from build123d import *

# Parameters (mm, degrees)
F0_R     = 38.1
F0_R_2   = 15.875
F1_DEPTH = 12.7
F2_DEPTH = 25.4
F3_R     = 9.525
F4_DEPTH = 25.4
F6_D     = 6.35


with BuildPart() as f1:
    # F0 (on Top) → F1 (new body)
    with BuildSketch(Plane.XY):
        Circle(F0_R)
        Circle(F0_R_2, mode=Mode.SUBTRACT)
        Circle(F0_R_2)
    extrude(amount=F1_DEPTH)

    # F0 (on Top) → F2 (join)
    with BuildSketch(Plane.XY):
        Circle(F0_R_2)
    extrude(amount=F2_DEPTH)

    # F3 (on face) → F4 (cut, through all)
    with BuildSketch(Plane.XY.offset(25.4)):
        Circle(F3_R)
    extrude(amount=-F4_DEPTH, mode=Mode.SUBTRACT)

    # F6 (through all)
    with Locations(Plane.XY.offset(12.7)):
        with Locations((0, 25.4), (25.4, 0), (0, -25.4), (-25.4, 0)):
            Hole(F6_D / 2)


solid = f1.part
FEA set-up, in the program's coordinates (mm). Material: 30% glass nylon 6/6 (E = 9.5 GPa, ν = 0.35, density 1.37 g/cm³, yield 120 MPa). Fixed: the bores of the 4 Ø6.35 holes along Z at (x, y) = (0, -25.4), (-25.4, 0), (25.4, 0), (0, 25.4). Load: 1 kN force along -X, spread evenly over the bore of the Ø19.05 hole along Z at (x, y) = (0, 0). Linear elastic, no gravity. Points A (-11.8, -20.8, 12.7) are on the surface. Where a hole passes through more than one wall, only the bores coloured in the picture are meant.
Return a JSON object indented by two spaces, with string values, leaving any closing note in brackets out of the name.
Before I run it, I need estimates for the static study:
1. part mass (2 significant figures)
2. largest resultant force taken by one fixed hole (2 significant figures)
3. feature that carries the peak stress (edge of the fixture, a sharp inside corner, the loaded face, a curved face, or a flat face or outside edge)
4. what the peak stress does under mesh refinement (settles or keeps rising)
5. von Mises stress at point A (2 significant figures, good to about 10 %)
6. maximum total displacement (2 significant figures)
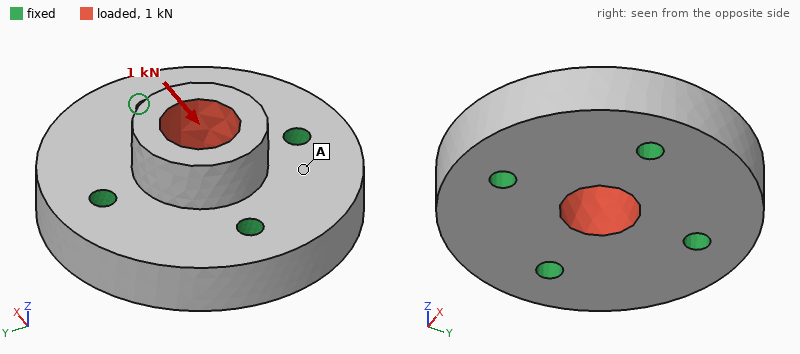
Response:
{
  "part mass": "81 g",
  "largest resultant force taken by one fixed hole": "340 N",
  "feature that carries the peak stress": "edge of the fixture",
  "what the peak stress does under mesh refinement": "keeps rising",
  "von Mises stress at point A": "0.44 MPa",
  "maximum total displacement": "8.9 µm"
}
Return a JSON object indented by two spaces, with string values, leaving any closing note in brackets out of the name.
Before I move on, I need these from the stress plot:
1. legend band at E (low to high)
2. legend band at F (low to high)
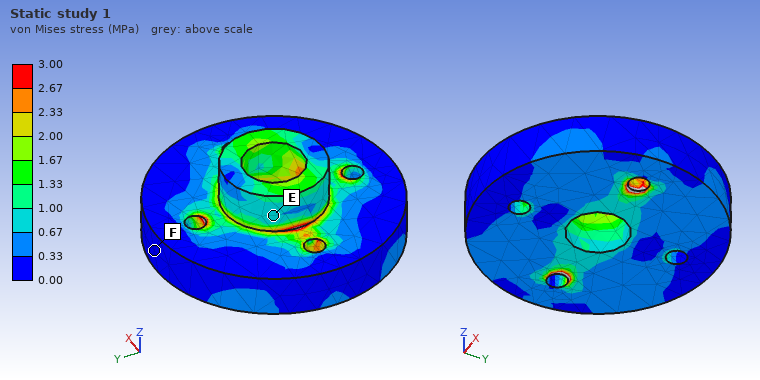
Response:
{
  "legend band at E": "0.67 to 1.00 MPa",
  "legend band at F": "0.00 to 0.33 MPa"
}
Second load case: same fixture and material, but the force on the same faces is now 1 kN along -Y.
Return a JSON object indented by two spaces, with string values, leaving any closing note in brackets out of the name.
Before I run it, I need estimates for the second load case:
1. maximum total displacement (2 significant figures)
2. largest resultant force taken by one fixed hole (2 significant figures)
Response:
{
  "maximum total displacement": "8.8 µm",
  "largest resultant force taken by one fixed hole": "340 N"
}
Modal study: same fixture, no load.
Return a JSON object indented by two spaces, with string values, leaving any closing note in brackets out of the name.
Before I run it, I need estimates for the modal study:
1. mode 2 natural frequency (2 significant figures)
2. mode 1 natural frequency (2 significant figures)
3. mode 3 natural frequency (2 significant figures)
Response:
{
  "mode 2 natural frequency": "11 kHz",
  "mode 1 natural frequency": "10 kHz",
  "mode 3 natural frequency": "11 kHz"
}
